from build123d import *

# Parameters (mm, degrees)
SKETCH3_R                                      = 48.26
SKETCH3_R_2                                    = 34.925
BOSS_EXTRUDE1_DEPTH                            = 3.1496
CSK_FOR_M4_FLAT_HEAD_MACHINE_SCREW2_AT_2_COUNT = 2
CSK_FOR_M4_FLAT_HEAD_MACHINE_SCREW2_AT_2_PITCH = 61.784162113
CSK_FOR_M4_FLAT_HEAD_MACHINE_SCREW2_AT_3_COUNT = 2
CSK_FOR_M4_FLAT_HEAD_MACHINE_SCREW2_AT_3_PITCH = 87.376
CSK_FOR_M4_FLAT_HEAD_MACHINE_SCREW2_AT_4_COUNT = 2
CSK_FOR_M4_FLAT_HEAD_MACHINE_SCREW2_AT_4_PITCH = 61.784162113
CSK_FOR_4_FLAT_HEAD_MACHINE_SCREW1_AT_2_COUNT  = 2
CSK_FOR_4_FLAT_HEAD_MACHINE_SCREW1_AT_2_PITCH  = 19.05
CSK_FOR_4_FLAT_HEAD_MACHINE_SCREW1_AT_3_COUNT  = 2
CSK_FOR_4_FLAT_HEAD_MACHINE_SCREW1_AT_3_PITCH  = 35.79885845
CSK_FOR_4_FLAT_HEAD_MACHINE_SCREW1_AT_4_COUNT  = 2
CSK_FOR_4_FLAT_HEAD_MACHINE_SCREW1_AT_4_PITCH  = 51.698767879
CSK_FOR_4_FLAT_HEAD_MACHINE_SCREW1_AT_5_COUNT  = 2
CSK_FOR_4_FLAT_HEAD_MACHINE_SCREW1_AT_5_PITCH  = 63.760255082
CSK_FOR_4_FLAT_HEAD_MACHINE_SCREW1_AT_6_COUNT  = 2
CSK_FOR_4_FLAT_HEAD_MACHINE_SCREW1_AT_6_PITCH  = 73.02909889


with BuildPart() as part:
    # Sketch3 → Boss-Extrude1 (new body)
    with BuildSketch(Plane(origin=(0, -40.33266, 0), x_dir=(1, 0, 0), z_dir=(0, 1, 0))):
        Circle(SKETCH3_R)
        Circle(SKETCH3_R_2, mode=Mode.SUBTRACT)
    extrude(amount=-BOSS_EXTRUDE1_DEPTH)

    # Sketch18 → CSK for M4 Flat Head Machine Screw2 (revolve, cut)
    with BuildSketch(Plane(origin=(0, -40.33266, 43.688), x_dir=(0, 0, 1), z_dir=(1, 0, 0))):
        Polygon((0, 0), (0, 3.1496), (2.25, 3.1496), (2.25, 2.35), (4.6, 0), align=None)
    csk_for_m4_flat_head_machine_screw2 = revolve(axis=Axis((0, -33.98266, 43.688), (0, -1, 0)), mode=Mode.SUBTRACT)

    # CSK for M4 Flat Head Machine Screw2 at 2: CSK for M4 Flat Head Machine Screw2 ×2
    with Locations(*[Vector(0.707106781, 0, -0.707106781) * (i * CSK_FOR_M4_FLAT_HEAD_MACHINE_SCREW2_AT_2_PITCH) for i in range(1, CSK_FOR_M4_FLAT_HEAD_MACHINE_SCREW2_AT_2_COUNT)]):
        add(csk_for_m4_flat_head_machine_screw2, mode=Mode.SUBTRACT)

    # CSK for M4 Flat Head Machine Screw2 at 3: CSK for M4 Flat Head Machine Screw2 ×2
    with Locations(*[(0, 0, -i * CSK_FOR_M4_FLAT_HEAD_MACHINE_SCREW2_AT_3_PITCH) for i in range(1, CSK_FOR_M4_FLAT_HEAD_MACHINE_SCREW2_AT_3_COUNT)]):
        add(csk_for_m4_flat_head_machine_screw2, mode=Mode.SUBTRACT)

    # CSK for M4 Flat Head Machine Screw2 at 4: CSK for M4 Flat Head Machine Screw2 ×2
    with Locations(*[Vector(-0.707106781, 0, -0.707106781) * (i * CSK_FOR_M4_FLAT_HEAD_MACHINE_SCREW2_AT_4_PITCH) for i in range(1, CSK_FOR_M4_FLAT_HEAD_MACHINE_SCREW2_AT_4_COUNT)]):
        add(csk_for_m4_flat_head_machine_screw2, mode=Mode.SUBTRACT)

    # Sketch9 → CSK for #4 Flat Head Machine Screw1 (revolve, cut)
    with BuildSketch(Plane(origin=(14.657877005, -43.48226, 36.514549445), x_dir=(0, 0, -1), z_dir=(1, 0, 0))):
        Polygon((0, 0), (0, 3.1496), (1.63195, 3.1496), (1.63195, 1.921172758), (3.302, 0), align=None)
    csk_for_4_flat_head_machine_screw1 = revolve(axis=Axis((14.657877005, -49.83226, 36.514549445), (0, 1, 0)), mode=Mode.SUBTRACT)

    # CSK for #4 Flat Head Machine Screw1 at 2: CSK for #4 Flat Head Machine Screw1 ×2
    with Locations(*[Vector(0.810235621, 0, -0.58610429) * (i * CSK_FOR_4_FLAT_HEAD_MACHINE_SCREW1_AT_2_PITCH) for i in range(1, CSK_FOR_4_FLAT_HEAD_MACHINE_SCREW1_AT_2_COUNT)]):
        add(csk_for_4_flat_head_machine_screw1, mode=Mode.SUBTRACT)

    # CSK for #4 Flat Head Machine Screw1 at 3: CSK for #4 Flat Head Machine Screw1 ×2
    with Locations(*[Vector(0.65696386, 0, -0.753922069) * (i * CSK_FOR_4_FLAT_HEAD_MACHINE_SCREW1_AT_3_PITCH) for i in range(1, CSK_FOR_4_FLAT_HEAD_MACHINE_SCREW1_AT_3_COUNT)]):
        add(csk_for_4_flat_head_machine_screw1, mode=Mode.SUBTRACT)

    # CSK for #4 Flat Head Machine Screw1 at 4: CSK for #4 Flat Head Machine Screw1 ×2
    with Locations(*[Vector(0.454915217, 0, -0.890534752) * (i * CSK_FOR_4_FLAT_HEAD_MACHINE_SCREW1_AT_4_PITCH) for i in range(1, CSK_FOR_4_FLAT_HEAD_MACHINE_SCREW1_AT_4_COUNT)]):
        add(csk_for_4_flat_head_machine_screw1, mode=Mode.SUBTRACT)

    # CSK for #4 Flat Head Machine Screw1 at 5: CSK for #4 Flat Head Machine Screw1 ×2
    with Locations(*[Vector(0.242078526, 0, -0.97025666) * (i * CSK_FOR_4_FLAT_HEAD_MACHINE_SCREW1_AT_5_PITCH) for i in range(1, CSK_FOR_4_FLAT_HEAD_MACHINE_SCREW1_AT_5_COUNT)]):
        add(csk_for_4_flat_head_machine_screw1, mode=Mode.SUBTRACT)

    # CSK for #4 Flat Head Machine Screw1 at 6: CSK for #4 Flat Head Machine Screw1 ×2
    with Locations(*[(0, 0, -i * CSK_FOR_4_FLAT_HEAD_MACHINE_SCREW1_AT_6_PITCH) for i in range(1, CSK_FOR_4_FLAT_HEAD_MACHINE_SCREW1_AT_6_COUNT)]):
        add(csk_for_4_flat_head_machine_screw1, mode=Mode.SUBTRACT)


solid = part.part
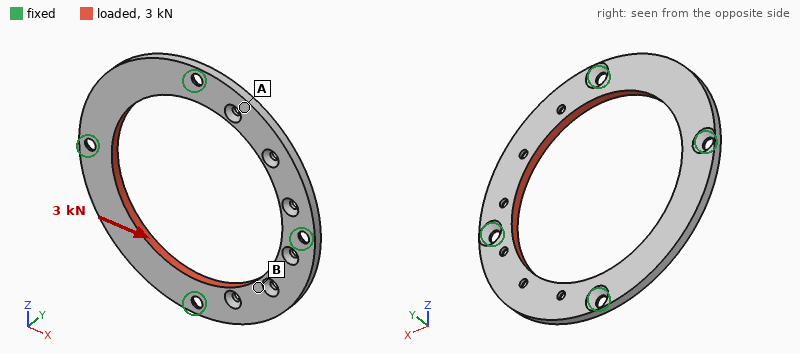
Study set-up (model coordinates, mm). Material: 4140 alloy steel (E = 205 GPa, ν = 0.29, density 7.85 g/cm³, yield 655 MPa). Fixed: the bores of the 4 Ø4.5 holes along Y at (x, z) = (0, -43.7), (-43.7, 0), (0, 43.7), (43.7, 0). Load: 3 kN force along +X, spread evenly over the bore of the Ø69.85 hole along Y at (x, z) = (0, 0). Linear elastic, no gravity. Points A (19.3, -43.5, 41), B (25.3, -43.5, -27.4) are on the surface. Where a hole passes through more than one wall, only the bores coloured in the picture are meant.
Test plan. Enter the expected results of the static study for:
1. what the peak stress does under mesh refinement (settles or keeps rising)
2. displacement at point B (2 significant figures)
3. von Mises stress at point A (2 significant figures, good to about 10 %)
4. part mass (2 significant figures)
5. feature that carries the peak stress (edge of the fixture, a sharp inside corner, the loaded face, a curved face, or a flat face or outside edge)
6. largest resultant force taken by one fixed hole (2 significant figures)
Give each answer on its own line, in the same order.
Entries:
keeps rising
6.3 µm
20 MPa
81 g
edge of the fixture
1000 N
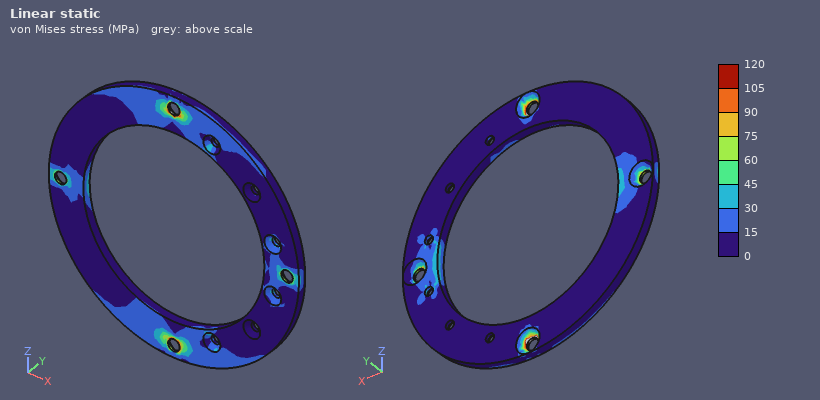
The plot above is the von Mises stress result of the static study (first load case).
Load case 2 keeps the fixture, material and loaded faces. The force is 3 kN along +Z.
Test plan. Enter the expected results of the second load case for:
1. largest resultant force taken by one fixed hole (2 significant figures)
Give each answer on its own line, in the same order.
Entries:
1000 N
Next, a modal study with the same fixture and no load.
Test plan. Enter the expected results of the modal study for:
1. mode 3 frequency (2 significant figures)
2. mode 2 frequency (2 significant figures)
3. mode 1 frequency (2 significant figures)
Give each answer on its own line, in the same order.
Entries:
2900 Hz
2900 Hz
2500 Hz
